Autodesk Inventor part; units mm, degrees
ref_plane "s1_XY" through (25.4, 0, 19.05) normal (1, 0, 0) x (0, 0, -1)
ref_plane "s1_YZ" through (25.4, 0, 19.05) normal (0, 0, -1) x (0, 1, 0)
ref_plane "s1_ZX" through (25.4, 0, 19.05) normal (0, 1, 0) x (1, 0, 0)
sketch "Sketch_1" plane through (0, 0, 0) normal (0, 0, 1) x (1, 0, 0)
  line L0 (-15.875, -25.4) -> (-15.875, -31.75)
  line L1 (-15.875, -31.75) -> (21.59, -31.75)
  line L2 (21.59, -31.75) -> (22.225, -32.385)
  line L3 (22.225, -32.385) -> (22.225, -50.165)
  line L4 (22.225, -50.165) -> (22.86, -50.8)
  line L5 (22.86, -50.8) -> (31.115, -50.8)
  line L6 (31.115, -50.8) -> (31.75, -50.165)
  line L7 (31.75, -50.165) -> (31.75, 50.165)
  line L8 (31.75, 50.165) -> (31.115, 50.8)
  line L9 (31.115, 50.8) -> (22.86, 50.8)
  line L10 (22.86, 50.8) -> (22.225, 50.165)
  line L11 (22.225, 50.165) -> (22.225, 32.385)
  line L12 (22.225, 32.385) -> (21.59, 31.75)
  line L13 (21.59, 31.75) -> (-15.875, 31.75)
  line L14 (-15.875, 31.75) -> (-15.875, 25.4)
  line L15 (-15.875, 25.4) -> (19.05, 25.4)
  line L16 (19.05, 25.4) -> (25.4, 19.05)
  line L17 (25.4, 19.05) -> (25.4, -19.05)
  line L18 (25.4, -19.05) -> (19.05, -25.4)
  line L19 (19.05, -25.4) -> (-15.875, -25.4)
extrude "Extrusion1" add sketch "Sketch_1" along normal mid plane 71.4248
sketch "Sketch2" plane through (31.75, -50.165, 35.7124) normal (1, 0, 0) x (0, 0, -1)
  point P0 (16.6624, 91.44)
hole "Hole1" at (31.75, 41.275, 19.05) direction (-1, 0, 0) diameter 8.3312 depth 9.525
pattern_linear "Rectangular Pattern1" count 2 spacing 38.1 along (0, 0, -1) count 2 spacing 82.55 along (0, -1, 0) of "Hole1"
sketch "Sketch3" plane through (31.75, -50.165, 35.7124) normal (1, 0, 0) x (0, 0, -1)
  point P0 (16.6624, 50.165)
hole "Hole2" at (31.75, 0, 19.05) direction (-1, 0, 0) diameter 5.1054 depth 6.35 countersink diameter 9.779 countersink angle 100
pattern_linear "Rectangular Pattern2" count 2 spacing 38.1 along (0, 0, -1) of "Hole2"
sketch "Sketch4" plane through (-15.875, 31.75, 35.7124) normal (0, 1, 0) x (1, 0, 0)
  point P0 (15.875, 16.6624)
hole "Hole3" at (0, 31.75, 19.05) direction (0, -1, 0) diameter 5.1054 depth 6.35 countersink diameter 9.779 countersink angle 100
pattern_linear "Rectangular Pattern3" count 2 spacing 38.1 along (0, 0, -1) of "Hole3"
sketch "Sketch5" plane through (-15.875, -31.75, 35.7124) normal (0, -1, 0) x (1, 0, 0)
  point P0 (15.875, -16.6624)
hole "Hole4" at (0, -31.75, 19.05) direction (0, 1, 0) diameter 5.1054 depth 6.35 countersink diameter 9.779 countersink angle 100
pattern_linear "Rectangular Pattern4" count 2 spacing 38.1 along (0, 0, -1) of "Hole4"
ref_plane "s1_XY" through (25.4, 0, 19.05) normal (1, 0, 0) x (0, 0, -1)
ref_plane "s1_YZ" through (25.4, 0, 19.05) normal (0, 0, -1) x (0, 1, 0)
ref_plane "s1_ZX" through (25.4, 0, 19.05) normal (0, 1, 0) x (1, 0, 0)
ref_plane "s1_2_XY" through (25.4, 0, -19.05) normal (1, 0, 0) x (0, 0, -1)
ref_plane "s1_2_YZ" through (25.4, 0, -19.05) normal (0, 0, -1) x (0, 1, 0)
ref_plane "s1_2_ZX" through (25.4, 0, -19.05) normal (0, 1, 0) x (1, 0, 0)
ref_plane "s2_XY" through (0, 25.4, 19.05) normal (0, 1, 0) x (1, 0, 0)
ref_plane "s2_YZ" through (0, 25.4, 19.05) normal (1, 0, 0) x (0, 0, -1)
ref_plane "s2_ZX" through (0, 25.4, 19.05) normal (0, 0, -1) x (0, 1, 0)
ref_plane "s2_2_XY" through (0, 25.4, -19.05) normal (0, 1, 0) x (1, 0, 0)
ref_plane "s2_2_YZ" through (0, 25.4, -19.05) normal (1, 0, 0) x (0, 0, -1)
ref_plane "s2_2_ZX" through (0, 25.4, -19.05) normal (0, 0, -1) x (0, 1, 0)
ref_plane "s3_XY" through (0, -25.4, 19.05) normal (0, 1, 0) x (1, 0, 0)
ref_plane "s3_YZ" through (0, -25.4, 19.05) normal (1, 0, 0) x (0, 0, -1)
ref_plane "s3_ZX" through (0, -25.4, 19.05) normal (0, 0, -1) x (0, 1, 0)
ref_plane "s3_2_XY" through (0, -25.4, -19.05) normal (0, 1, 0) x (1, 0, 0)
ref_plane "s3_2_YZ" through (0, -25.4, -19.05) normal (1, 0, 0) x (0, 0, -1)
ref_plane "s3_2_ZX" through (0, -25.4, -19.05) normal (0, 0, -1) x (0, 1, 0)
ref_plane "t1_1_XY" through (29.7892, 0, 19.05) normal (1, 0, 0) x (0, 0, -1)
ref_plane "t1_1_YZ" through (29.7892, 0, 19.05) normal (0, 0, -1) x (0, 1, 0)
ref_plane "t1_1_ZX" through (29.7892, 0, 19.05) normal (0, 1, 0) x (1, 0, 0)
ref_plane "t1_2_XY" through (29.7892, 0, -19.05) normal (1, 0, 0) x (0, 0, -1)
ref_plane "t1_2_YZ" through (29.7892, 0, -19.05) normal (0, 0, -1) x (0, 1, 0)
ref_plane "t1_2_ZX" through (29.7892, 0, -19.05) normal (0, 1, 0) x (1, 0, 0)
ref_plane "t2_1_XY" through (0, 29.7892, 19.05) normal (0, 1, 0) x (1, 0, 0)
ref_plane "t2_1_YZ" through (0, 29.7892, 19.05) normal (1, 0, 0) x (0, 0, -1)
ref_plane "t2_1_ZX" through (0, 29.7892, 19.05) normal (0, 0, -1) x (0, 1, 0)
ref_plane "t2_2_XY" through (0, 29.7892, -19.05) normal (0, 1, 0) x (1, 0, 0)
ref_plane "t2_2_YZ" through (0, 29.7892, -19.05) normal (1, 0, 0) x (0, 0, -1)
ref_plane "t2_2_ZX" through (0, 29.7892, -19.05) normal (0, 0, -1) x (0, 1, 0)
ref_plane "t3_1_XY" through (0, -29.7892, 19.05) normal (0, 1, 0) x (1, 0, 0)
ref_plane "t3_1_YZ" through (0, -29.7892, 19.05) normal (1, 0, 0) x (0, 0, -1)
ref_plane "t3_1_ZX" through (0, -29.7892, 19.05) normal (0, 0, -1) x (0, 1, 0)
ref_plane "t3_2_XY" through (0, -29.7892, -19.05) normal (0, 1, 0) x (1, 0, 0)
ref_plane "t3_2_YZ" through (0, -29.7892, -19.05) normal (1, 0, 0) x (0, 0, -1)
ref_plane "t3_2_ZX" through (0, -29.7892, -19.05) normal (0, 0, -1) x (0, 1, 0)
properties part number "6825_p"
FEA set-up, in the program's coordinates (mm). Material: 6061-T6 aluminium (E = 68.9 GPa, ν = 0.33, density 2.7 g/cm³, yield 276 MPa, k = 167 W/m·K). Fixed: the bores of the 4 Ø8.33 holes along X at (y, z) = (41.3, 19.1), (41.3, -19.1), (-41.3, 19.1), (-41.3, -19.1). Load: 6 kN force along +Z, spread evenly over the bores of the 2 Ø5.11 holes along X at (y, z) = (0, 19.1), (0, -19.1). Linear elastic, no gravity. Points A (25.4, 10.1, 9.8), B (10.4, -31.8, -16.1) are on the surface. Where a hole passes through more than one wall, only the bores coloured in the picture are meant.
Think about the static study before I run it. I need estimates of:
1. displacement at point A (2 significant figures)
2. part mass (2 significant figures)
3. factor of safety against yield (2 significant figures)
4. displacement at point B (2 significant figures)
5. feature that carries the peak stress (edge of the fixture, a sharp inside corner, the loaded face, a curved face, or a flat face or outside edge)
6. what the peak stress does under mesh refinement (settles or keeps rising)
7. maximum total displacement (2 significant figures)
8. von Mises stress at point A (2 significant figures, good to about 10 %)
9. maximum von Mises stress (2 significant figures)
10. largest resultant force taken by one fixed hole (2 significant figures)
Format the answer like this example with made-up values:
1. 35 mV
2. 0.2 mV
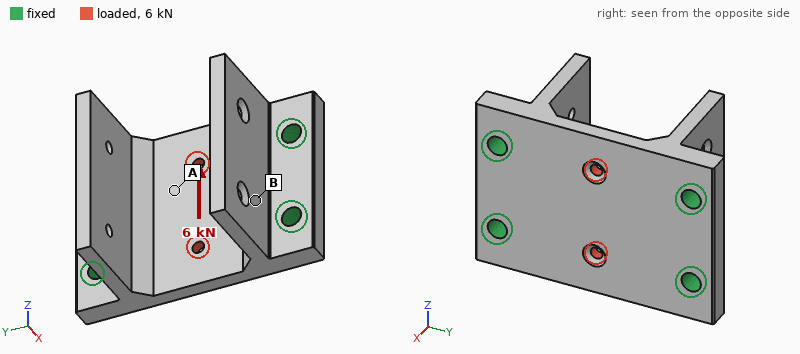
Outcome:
1. 8.6 µm
2. 250 g
3. 3.7
4. 2.6 µm
5. the loaded face
6. settles
7. 15 µm
8. 16 MPa
9. 75 MPa
10. 1.8 kN
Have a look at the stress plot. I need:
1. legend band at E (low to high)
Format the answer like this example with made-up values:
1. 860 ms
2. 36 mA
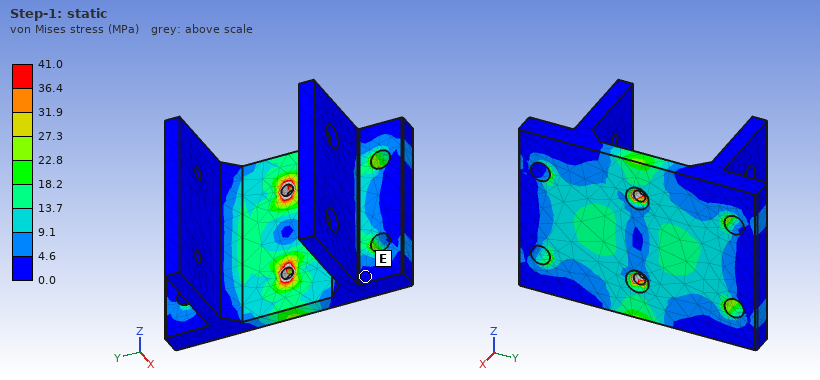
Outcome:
1. 0.0 to 4.6 MPa
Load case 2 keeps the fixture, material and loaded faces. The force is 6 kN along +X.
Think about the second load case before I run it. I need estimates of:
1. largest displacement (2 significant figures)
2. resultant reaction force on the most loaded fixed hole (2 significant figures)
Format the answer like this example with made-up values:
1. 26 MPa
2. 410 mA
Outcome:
1. 0.10 mm
2. 2.1 kN
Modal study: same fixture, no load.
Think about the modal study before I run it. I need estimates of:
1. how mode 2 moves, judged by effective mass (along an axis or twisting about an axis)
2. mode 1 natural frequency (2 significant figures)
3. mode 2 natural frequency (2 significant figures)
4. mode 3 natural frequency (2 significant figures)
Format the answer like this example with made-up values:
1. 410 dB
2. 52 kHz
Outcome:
1. along Y
2. 2900 Hz
3. 3300 Hz
4. 4700 Hz
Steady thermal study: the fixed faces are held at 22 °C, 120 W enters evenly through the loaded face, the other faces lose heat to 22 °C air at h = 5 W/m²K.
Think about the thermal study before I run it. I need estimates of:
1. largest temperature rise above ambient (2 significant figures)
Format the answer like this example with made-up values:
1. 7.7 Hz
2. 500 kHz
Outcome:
1. 38 K
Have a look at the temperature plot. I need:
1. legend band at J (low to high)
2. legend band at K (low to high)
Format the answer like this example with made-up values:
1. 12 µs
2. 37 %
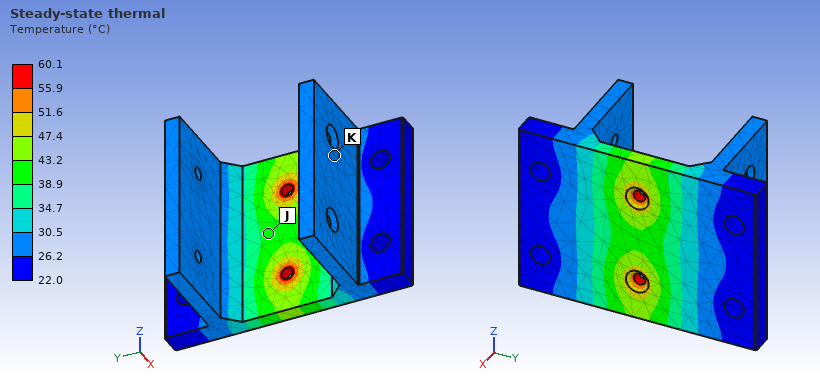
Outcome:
1. 38.9 to 43.2 °C
2. 26.2 to 30.5 °C
